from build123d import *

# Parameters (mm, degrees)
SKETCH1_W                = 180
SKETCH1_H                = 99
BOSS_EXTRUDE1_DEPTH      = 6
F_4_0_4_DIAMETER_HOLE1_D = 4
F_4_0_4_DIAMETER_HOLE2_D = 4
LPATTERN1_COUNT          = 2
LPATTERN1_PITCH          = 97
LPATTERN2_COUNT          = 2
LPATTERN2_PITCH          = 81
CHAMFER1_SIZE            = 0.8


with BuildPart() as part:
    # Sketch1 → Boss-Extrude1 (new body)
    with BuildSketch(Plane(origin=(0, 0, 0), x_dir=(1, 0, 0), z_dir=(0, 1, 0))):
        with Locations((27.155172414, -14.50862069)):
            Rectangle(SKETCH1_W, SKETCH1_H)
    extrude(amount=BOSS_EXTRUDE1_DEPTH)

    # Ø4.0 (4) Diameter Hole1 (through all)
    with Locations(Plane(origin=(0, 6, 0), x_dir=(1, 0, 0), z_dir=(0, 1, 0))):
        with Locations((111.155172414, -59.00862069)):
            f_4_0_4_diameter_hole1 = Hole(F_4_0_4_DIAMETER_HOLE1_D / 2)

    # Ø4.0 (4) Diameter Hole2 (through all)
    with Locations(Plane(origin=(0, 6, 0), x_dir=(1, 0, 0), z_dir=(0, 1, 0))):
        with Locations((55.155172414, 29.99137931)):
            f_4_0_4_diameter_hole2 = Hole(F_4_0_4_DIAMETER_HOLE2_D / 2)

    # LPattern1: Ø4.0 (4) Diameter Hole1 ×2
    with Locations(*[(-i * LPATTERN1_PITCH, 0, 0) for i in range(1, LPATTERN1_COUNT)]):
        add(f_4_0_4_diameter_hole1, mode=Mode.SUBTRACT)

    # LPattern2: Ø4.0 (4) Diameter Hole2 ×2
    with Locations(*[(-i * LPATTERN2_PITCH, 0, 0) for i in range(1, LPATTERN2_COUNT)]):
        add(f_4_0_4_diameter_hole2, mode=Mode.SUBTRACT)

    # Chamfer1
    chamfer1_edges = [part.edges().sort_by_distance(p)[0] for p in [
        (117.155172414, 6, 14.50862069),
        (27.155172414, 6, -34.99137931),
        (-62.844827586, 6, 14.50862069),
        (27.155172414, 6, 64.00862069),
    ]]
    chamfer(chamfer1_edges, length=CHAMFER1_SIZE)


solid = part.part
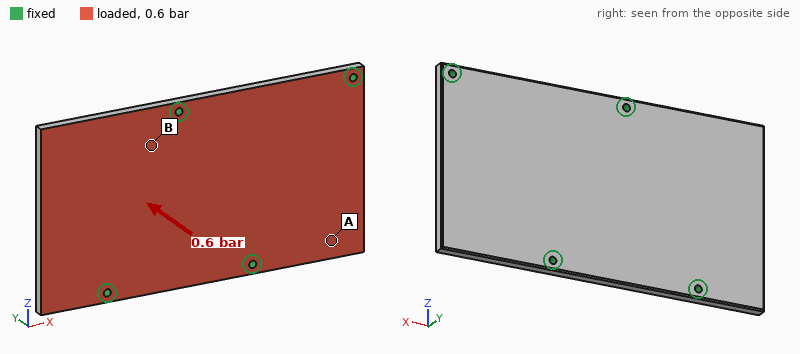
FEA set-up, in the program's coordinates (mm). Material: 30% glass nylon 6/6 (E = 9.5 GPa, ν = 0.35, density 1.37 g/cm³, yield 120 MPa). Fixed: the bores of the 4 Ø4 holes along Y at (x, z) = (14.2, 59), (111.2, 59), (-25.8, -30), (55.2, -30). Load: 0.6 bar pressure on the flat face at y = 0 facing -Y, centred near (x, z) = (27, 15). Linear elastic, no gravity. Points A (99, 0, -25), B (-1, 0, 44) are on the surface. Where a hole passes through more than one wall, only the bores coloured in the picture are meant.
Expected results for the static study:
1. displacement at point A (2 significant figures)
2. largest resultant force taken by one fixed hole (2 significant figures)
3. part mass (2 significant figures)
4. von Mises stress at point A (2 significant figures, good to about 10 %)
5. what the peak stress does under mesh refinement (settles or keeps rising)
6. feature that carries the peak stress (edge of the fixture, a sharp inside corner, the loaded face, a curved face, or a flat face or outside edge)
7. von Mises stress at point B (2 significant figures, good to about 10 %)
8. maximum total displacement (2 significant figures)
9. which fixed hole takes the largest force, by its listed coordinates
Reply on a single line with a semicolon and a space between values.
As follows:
0.31 mm; 340 N; 150 g; 4.1 MPa; keeps rising; edge of the fixture; 11 MPa; 1.1 mm; (14.2, 59)
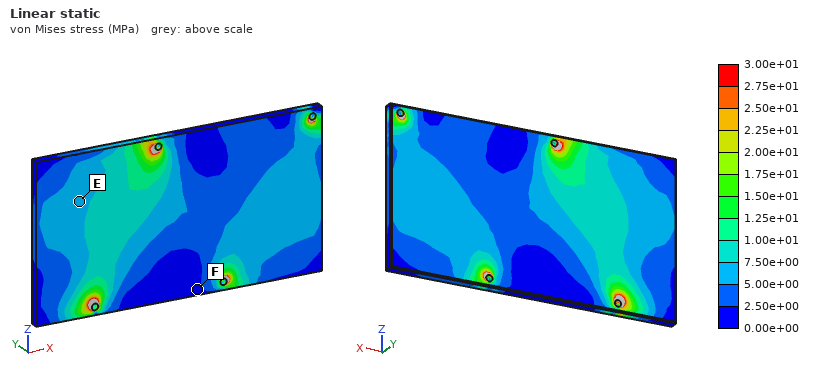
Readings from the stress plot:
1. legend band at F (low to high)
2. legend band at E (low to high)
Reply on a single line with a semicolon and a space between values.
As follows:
0.00e+00 to 2.50e+00 MPa; 5.00e+00 to 7.50e+00 MPa
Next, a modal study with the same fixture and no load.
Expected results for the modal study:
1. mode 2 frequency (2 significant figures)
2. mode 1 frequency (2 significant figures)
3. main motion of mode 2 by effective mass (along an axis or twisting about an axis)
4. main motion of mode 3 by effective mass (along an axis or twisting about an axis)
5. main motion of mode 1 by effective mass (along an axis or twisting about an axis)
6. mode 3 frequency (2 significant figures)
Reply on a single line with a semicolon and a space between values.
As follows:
820 Hz; 570 Hz; along Y; along Y; along Y; 1300 Hz
